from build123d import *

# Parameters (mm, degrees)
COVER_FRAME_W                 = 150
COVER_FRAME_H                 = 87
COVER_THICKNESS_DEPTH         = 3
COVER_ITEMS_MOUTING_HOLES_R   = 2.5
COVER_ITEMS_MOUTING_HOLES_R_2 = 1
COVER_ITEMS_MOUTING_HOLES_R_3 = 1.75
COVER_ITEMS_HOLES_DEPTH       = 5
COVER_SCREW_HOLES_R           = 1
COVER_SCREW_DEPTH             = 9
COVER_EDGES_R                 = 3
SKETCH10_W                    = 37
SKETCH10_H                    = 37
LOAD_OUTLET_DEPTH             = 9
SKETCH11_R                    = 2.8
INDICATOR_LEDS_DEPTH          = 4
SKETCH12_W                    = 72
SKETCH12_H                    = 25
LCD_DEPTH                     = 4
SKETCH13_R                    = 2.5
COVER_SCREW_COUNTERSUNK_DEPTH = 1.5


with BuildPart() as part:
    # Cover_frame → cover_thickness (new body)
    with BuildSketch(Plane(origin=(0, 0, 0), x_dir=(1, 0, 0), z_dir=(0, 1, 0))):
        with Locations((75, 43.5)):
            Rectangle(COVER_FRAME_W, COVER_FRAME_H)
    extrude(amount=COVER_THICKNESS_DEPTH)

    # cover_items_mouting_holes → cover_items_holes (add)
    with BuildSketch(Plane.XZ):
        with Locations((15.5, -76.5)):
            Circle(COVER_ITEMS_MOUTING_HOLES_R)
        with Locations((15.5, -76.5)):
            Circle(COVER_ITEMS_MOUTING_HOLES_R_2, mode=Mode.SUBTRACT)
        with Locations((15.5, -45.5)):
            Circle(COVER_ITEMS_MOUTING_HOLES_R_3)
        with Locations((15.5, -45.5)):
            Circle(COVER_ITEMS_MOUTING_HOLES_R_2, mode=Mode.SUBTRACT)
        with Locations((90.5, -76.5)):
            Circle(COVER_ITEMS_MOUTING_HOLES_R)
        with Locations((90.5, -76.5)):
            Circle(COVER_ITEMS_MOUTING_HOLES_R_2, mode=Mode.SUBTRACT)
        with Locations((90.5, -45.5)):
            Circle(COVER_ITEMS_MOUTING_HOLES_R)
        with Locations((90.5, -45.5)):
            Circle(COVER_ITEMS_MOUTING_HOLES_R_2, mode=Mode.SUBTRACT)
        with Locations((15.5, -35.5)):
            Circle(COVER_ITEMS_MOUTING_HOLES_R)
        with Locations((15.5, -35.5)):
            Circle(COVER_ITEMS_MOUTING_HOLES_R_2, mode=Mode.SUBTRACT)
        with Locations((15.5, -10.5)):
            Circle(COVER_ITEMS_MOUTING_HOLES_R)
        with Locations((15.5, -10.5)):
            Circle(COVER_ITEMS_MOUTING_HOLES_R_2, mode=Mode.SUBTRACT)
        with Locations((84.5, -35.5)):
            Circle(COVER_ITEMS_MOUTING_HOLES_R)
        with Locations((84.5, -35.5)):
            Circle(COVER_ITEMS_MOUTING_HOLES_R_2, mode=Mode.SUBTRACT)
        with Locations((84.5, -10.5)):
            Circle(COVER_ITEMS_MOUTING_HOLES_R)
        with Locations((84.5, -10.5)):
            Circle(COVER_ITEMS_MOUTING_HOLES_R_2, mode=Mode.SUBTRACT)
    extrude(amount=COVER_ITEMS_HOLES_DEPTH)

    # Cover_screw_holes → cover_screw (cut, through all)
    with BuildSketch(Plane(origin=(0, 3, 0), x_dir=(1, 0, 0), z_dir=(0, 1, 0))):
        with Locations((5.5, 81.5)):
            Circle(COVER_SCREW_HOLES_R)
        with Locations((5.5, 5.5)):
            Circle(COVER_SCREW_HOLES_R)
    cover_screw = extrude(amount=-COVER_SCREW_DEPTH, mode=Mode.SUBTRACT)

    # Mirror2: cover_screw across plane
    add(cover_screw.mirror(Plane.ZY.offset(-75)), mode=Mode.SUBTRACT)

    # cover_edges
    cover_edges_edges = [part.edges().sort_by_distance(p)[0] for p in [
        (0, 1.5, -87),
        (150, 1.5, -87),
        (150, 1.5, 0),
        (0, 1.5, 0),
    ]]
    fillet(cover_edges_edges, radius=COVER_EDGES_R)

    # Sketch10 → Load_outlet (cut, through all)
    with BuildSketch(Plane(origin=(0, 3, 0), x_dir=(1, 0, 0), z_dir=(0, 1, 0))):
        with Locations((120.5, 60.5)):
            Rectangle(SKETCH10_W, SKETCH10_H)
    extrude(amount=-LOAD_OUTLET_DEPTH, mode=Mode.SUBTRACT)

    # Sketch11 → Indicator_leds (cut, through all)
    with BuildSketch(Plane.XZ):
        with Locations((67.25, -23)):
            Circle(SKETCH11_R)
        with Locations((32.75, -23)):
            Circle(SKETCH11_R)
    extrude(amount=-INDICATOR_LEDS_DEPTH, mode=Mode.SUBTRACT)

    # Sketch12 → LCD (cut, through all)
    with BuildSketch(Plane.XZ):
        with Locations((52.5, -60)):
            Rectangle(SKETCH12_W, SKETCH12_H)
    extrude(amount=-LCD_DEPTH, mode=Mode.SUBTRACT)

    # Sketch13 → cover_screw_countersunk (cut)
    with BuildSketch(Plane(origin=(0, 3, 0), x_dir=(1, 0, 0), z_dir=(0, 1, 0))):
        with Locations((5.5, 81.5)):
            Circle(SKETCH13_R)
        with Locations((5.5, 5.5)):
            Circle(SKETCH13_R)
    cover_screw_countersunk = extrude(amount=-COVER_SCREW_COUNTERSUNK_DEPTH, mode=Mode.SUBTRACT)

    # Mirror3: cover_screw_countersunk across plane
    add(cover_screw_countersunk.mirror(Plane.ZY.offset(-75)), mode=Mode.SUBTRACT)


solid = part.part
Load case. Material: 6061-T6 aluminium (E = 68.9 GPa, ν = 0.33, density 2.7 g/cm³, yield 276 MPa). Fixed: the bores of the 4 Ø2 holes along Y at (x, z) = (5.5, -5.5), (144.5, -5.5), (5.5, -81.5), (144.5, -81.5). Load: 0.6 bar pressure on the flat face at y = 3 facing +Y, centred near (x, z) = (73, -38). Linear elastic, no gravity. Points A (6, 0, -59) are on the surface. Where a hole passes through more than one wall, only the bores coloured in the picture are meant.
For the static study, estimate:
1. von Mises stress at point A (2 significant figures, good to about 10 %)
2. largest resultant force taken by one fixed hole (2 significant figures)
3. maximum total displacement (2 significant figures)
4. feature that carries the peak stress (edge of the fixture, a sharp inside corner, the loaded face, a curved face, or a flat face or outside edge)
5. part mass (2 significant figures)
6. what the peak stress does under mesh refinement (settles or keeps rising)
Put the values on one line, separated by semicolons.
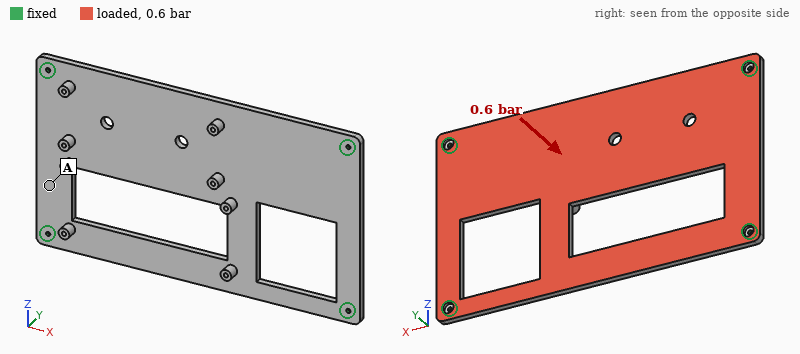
25 MPa; 480 N; 0.91 mm; edge of the fixture; 81 g; keeps rising
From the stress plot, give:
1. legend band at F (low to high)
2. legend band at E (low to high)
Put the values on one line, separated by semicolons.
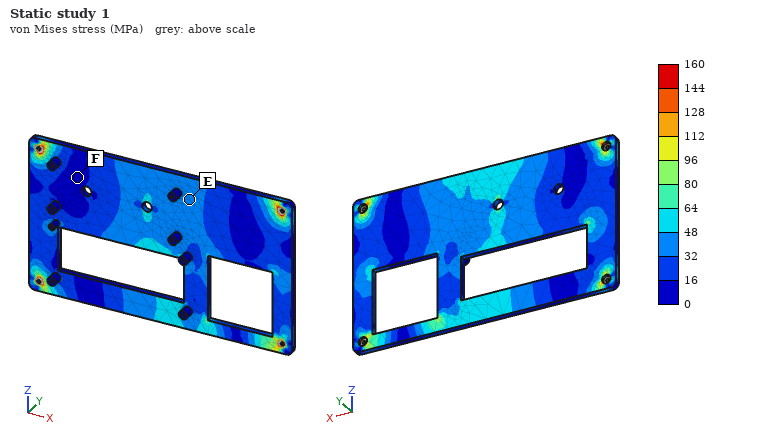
0 to 16 MPa; 32 to 48 MPa
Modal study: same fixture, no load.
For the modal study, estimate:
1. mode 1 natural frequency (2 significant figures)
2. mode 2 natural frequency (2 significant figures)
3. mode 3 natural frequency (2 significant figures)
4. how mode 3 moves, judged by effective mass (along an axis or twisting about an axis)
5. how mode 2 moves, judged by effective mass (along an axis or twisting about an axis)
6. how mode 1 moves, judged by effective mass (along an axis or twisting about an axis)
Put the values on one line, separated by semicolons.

530 Hz; 880 Hz; 1400 Hz; twisting about Z; twisting about X; along Y
